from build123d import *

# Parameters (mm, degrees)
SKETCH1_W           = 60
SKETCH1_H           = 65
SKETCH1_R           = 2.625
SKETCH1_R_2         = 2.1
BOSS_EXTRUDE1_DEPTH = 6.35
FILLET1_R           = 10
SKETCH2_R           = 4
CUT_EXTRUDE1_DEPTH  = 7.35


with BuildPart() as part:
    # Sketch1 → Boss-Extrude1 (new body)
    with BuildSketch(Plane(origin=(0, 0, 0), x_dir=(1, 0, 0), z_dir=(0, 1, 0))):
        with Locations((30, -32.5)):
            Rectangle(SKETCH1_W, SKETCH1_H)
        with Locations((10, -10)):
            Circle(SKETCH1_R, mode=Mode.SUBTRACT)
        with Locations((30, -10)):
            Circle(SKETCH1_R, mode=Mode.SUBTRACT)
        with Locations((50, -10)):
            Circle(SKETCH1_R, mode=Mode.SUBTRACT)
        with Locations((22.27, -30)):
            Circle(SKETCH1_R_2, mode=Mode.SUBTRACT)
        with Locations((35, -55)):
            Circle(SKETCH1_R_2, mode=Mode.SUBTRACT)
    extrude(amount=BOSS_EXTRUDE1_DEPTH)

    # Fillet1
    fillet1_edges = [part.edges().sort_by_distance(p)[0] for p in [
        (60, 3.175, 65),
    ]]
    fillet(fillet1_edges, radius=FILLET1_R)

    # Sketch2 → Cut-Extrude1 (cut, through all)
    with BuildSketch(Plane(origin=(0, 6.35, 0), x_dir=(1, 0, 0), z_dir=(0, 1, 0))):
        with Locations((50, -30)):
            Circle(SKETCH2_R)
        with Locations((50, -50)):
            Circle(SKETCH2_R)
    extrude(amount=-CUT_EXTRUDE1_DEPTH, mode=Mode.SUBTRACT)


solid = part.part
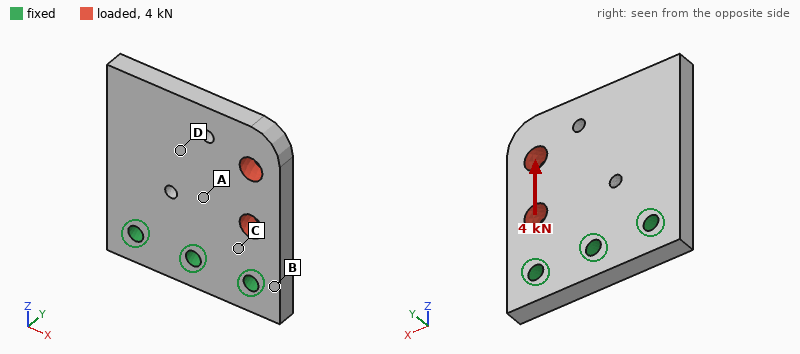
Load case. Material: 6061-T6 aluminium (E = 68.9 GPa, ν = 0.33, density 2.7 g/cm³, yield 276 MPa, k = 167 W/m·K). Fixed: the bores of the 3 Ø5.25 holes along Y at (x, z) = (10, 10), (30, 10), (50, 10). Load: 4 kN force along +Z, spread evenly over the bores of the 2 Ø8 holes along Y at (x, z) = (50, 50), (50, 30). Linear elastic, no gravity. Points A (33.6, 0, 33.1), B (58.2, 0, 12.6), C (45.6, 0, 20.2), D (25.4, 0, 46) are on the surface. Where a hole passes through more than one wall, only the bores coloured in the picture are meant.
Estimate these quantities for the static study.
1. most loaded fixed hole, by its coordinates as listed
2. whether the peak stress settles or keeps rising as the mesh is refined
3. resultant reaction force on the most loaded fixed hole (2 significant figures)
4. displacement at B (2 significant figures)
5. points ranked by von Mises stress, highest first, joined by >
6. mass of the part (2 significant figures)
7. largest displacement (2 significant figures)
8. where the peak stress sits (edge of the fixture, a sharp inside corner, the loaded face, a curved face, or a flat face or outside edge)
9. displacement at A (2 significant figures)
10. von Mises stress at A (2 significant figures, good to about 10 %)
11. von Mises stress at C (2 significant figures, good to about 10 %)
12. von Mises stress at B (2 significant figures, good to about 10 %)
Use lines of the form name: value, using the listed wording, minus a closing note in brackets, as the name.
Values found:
most loaded fixed hole, by its coordinates as listed: (50, 10)
whether the peak stress settles or keeps rising as the mesh is refined: keeps rising
resultant reaction force on the most loaded fixed hole: 3.3 kN
displacement at B: 4.9 µm
points ranked by von Mises stress, highest first, joined by >: C > B > A > D
mass of the part: 63 g
largest displacement: 23 µm
where the peak stress sits: edge of the fixture
displacement at A: 5.3 µm
von Mises stress at A: 9.0 MPa
von Mises stress at C: 26 MPa
von Mises stress at B: 17 MPa
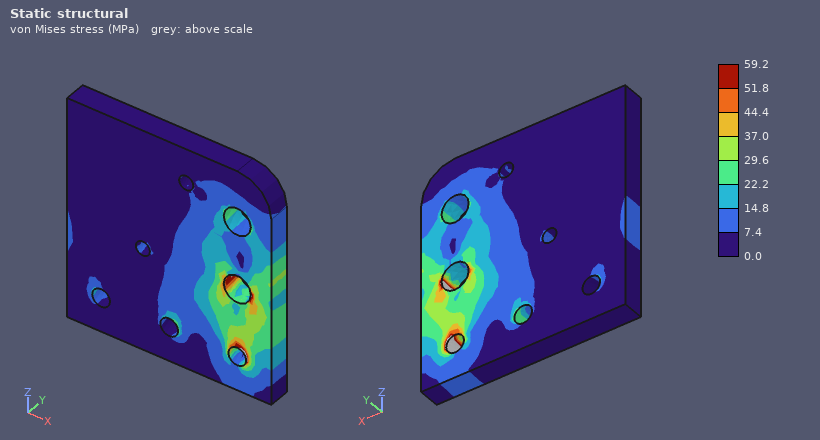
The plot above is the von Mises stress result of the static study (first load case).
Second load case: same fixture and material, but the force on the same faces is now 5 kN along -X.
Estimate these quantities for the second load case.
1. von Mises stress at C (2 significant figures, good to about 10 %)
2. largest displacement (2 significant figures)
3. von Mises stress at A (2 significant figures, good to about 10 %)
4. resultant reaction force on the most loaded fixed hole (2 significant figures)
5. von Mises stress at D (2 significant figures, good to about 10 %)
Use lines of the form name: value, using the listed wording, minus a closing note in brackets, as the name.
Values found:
von Mises stress at C: 47 MPa
largest displacement: 42 µm
von Mises stress at A: 29 MPa
resultant reaction force on the most loaded fixed hole: 3.9 kN
von Mises stress at D: 15 MPa
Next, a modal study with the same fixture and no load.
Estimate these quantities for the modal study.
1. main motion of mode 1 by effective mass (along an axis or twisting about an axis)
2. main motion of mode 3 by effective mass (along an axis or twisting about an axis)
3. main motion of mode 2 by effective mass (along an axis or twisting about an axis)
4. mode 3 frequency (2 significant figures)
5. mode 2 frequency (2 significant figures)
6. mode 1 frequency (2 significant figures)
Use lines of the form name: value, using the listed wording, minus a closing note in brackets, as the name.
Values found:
main motion of mode 1 by effective mass: along Y
main motion of mode 3 by effective mass: along X
main motion of mode 2 by effective mass: twisting about Z
mode 3 frequency: 9100 Hz
mode 2 frequency: 3900 Hz
mode 1 frequency: 1800 Hz
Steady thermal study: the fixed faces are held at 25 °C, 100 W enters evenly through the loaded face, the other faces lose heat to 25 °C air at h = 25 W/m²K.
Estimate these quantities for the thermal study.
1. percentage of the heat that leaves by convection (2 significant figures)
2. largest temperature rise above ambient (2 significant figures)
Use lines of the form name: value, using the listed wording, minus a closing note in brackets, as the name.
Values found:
percentage of the heat that leaves by convection: 6.3 %
largest temperature rise above ambient: 74 K
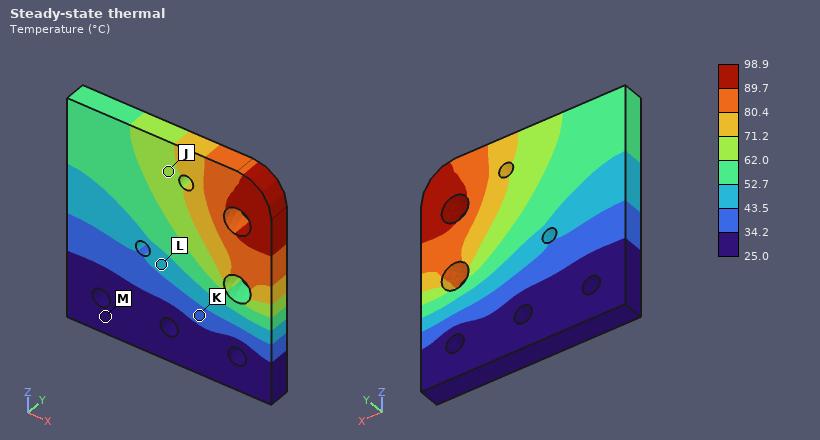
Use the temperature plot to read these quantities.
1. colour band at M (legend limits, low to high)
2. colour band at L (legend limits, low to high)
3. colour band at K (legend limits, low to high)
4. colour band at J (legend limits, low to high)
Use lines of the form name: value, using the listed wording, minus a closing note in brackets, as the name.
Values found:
colour band at M: 25.0 to 34.2 °C
colour band at L: 43.5 to 52.7 °C
colour band at K: 34.2 to 43.5 °C
colour band at J: 62.0 to 71.2 °C
